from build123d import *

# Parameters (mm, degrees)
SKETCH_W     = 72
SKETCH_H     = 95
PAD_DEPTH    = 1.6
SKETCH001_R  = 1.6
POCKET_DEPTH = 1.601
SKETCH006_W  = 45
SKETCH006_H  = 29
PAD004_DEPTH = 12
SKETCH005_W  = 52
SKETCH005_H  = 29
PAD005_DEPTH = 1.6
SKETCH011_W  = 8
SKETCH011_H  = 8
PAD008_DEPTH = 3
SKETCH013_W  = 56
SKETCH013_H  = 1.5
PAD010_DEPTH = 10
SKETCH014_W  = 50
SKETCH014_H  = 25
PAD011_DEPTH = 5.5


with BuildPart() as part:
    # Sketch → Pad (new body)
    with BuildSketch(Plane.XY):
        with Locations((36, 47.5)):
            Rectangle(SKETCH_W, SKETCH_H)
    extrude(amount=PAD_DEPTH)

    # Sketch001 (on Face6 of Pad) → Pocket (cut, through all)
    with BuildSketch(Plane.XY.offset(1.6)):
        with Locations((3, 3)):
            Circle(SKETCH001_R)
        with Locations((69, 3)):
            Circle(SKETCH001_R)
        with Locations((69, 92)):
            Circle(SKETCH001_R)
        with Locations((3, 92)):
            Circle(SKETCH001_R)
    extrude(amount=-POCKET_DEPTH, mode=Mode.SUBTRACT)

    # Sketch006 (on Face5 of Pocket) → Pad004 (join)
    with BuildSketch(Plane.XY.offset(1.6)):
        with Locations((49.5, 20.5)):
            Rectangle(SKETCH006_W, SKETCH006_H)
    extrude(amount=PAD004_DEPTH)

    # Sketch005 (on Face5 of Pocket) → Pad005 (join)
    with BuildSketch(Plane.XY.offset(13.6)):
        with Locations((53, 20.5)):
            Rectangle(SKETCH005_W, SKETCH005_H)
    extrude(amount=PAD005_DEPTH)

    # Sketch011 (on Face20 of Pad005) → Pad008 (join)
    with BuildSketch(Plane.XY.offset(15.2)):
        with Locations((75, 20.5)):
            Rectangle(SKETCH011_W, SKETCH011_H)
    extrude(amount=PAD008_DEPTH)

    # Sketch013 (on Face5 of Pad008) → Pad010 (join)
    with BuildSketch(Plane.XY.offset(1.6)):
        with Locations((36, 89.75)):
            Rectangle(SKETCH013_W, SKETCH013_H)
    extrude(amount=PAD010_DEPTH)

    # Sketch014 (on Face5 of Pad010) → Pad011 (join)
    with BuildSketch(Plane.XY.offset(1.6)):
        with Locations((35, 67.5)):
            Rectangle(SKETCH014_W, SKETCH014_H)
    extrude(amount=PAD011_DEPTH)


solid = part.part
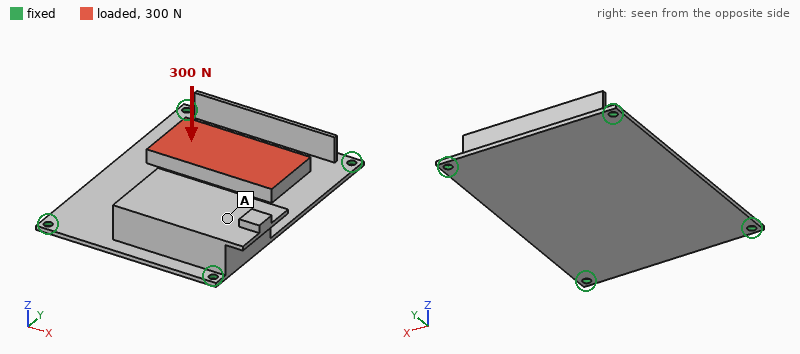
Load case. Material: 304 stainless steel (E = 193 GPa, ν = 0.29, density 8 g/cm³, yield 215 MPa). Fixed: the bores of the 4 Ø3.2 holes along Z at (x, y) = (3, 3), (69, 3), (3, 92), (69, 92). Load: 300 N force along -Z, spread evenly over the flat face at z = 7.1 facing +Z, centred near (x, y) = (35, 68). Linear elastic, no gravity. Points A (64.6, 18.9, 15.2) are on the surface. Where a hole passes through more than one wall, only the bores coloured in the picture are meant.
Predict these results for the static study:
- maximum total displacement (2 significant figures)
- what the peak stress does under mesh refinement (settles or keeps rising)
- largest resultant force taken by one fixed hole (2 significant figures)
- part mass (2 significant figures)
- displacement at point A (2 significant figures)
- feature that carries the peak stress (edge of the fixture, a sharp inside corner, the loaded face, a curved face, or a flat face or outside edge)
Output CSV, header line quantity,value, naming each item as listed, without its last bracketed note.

quantity,value
maximum total displacement,0.15 mm
what the peak stress does under mesh refinement,keeps rising
largest resultant force taken by one fixed hole,150 N
part mass,290 g
displacement at point A,0.076 mm
feature that carries the peak stress,edge of the fixture
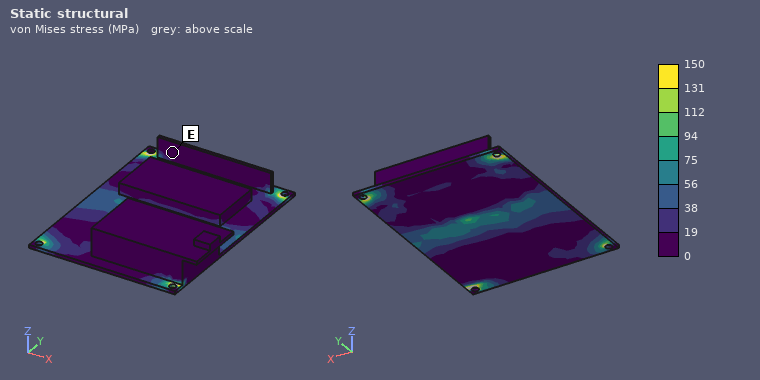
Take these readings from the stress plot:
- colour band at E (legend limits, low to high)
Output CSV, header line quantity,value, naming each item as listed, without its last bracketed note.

quantity,value
colour band at E,0 to 19 MPa
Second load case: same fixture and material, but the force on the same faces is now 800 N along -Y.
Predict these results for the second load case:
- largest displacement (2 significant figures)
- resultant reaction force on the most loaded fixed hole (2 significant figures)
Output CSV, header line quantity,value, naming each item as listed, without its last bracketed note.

quantity,value
largest displacement,0.12 mm
resultant reaction force on the most loaded fixed hole,260 N
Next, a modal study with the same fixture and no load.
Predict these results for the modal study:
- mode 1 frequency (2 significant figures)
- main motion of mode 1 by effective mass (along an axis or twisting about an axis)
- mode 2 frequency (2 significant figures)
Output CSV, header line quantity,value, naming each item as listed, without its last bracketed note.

quantity,value
mode 1 frequency,540 Hz
main motion of mode 1 by effective mass,along Z
mode 2 frequency,1300 Hz
